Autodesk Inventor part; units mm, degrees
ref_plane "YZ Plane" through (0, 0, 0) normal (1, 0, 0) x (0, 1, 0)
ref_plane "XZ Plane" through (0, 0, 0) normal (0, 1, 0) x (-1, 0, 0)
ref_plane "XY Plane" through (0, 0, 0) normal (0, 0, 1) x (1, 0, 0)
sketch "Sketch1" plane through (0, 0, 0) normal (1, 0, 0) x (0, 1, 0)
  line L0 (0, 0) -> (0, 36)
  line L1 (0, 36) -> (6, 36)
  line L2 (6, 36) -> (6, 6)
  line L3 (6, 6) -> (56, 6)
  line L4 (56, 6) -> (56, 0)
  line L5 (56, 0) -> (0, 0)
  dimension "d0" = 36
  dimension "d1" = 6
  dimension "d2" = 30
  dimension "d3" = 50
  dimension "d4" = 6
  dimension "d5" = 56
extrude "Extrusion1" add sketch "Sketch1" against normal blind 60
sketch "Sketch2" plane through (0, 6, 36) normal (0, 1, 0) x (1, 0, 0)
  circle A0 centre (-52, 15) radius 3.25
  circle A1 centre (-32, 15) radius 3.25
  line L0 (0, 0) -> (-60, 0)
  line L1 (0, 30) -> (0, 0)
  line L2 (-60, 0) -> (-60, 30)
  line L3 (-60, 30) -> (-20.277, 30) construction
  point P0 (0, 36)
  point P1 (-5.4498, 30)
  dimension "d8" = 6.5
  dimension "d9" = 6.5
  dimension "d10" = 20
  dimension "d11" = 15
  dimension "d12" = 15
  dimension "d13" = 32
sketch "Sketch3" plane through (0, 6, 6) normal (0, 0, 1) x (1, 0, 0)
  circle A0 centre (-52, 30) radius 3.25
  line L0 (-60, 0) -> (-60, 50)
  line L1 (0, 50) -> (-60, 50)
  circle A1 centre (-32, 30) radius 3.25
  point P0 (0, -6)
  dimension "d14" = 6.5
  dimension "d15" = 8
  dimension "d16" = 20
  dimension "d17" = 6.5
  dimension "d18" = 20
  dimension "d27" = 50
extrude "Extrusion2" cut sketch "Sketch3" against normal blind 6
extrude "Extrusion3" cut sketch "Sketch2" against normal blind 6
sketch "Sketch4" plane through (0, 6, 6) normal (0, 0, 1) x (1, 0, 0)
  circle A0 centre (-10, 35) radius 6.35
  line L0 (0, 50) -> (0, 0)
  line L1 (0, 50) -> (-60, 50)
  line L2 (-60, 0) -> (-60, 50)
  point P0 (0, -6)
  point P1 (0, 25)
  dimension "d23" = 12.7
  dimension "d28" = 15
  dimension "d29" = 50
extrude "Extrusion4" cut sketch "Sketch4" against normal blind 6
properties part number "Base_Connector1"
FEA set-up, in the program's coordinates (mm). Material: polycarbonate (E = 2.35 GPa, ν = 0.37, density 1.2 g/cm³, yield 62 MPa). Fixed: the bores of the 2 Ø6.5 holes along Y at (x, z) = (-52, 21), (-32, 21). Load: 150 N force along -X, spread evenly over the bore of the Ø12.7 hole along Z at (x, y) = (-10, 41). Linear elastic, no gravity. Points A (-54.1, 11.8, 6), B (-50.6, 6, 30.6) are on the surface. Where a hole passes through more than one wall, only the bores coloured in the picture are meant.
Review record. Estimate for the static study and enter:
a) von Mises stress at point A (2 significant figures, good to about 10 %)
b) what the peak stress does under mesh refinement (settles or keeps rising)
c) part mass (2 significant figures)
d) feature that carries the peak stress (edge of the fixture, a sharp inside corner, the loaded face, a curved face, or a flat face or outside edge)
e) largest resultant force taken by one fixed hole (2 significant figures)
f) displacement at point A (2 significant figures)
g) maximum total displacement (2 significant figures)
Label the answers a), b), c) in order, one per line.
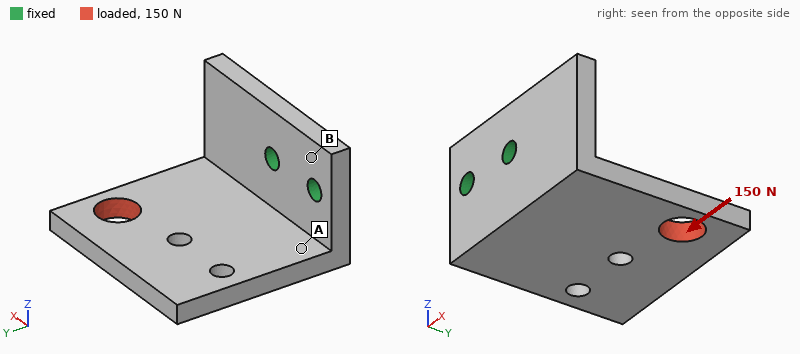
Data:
a) 6.6 MPa
b) keeps rising
c) 35 g
d) edge of the fixture
e) 240 N
f) 0.22 mm
g) 0.99 mm
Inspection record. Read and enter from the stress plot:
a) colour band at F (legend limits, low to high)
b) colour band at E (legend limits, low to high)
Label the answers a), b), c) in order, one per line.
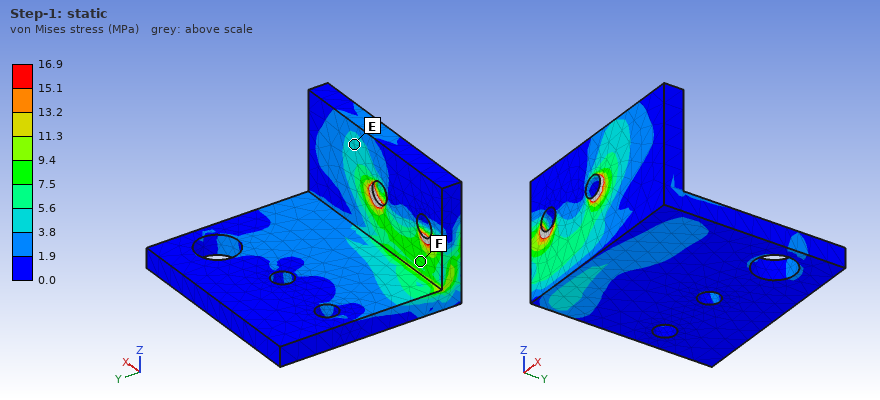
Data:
a) 7.5 to 9.4 MPa
b) 3.8 to 5.6 MPa
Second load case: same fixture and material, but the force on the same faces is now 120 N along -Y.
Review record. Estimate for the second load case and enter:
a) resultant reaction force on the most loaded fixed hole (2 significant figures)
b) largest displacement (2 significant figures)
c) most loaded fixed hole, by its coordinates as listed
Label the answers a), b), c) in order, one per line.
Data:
a) 190 N
b) 0.93 mm
c) (-32, 21)
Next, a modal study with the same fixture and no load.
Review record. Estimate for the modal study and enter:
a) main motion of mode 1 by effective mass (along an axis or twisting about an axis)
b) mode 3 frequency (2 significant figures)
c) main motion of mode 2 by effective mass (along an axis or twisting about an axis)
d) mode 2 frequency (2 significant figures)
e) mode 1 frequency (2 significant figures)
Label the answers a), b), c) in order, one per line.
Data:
a) along Z
b) 960 Hz
c) along X
d) 600 Hz
e) 330 Hz
